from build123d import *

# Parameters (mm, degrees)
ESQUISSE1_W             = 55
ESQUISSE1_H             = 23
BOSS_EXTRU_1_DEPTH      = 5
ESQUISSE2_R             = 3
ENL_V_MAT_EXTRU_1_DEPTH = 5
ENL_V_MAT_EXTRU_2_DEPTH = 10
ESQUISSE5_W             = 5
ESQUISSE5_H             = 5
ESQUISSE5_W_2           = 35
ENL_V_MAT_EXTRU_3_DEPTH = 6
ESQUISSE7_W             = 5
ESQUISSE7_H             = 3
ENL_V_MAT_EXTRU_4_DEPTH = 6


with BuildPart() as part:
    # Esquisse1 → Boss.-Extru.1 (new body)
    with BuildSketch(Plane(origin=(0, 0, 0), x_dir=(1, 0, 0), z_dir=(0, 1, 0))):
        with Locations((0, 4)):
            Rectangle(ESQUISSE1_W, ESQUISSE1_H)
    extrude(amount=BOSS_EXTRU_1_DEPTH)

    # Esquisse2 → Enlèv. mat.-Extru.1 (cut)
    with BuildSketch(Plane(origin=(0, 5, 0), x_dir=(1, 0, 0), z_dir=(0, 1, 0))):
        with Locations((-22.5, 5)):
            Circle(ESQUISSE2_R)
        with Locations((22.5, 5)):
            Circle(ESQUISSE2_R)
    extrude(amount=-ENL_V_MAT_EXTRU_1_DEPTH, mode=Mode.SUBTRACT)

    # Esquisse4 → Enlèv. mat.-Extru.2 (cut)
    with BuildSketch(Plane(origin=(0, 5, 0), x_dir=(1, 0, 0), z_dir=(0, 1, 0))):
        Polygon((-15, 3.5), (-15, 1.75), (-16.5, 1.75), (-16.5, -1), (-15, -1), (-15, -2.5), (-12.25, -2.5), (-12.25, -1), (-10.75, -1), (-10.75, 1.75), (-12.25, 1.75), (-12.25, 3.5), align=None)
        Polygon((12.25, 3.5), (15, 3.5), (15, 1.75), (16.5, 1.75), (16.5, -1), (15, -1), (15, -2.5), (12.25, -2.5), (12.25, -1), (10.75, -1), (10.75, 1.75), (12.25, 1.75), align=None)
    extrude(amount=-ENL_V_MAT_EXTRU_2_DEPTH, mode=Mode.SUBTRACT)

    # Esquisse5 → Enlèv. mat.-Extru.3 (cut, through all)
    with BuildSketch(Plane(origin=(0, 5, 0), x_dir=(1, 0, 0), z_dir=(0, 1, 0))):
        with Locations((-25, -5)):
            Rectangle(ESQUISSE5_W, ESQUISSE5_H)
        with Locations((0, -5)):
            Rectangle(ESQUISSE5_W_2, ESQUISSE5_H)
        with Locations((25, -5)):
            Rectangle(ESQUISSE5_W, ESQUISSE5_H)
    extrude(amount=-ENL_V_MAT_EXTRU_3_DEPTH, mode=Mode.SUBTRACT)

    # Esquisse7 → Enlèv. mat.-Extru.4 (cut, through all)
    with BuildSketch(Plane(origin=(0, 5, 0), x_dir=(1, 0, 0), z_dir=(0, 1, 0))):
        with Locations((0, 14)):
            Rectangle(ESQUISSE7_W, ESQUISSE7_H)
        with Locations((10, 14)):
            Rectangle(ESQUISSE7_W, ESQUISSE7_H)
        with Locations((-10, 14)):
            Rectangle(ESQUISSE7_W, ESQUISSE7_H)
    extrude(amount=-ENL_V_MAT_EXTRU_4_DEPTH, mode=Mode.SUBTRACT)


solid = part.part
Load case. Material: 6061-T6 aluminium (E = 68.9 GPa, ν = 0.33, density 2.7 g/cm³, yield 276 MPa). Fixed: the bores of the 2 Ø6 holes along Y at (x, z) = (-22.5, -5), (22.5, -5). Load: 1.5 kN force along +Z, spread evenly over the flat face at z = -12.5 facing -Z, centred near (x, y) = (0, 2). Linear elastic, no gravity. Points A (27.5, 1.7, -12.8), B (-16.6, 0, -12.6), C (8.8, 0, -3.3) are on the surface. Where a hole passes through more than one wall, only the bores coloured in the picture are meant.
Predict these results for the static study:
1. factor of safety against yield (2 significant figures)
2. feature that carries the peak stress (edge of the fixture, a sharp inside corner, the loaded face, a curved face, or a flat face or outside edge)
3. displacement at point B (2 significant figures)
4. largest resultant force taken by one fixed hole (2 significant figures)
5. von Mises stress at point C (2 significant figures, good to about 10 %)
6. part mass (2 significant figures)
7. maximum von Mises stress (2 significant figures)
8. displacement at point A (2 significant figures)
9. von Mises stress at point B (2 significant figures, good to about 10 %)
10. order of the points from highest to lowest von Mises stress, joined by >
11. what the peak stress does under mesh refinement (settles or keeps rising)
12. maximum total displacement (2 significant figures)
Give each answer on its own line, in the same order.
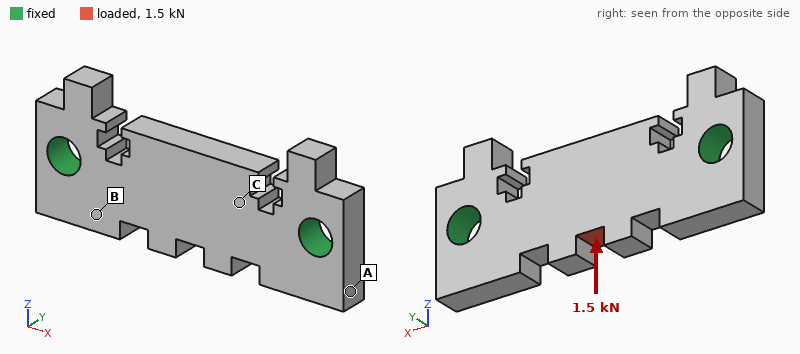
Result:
3.3
the loaded face
6.6 µm
750 N
22 MPa
12 g
83 MPa
4.6 µm
14 MPa
C > B > A
settles
24 µm
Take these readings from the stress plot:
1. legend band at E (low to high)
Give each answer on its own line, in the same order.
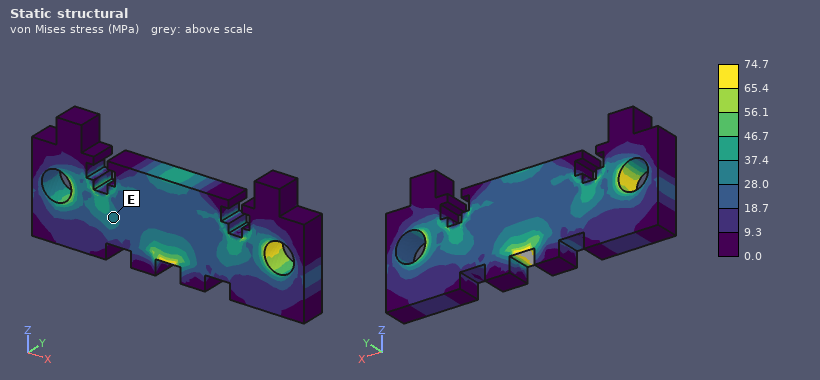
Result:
28.0 to 37.4 MPa
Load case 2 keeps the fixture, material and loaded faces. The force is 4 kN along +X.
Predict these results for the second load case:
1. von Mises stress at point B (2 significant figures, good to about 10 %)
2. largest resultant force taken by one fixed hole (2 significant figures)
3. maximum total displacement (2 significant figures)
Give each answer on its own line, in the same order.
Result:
16 MPa
2.1 kN
25 µm
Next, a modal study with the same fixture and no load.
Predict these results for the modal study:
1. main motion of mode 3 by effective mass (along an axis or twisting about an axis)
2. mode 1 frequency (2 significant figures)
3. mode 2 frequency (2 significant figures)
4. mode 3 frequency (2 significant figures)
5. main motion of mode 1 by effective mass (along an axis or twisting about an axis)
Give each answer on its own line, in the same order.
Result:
along Z
12 kHz
16 kHz
21 kHz
along Y
